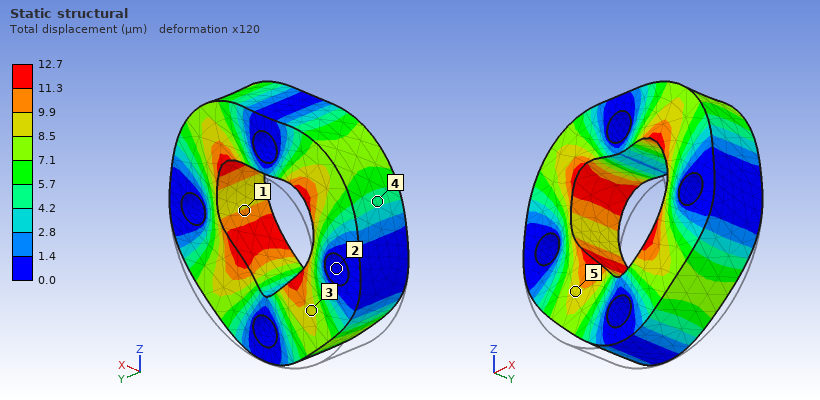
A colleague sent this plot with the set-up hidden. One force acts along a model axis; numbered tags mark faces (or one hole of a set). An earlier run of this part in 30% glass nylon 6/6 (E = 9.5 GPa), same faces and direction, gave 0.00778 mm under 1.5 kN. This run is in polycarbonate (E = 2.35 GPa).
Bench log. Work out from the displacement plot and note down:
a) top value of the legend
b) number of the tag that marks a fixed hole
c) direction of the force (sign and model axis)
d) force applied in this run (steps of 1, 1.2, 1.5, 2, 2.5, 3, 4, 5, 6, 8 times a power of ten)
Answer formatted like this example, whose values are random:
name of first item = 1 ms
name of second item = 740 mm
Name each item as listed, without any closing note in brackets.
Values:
top value of the legend = 12.7 µm
number of the tag that marks a fixed hole = 2
direction of the force = +Z
force applied in this run = 600 N
